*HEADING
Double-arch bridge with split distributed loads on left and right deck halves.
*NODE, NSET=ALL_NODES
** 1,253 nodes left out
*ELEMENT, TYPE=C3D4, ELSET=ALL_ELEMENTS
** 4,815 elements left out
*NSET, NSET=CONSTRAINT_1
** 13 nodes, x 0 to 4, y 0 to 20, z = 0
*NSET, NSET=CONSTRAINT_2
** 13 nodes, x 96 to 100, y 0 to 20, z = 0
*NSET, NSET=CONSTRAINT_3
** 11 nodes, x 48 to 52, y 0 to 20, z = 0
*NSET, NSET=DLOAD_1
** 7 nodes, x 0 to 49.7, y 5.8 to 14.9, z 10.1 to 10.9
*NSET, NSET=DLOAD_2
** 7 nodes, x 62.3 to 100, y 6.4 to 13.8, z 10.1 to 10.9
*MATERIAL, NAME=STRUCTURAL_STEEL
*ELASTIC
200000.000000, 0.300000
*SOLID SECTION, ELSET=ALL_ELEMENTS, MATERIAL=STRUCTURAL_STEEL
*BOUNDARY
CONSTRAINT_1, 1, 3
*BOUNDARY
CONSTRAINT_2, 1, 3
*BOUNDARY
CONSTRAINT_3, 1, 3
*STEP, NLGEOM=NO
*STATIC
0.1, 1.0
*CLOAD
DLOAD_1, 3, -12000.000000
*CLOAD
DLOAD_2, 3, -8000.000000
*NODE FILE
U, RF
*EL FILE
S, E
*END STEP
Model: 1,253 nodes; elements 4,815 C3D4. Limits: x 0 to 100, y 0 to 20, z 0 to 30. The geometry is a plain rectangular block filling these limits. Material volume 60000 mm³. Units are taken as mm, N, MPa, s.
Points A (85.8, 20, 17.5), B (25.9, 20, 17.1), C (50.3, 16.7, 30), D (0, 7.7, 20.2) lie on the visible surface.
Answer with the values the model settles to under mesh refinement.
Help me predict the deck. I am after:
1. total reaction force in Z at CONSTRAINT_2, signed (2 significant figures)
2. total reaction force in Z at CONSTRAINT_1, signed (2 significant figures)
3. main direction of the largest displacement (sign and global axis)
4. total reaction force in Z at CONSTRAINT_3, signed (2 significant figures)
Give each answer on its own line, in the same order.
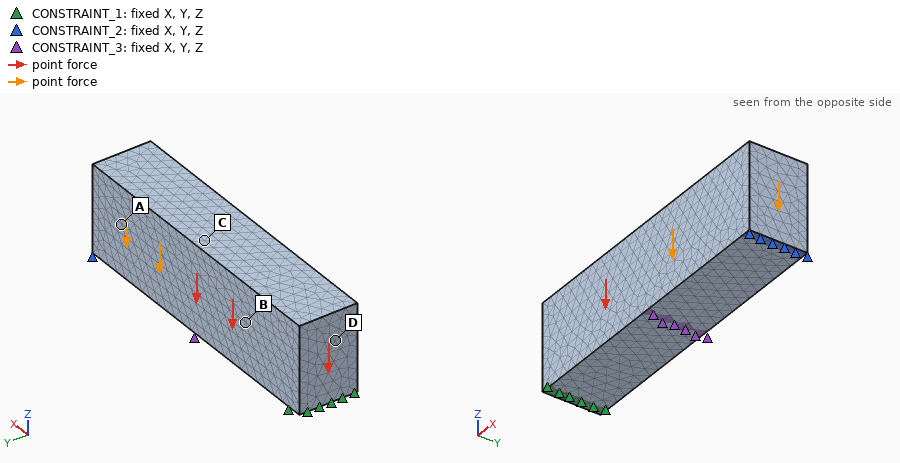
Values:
38000 N
56000 N
-Z
46000 N
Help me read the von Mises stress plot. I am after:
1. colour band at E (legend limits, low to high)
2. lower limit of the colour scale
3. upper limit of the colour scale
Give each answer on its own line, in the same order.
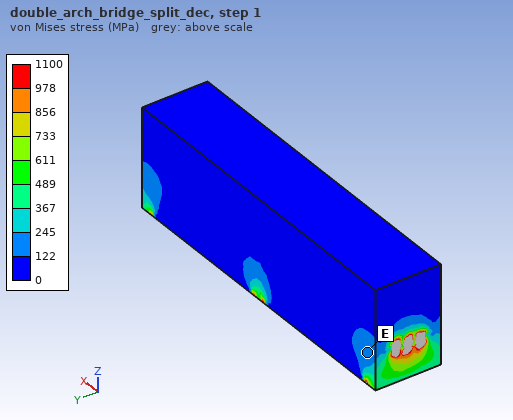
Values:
122 to 245 MPa
0 MPa
1100 MPa
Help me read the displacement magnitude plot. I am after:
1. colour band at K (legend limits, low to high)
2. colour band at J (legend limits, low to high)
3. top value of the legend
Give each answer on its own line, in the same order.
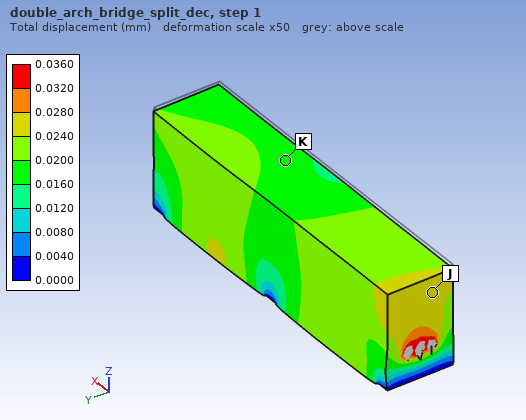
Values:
0.0160 to 0.0200 mm
0.0240 to 0.0280 mm
0.0360 mm
